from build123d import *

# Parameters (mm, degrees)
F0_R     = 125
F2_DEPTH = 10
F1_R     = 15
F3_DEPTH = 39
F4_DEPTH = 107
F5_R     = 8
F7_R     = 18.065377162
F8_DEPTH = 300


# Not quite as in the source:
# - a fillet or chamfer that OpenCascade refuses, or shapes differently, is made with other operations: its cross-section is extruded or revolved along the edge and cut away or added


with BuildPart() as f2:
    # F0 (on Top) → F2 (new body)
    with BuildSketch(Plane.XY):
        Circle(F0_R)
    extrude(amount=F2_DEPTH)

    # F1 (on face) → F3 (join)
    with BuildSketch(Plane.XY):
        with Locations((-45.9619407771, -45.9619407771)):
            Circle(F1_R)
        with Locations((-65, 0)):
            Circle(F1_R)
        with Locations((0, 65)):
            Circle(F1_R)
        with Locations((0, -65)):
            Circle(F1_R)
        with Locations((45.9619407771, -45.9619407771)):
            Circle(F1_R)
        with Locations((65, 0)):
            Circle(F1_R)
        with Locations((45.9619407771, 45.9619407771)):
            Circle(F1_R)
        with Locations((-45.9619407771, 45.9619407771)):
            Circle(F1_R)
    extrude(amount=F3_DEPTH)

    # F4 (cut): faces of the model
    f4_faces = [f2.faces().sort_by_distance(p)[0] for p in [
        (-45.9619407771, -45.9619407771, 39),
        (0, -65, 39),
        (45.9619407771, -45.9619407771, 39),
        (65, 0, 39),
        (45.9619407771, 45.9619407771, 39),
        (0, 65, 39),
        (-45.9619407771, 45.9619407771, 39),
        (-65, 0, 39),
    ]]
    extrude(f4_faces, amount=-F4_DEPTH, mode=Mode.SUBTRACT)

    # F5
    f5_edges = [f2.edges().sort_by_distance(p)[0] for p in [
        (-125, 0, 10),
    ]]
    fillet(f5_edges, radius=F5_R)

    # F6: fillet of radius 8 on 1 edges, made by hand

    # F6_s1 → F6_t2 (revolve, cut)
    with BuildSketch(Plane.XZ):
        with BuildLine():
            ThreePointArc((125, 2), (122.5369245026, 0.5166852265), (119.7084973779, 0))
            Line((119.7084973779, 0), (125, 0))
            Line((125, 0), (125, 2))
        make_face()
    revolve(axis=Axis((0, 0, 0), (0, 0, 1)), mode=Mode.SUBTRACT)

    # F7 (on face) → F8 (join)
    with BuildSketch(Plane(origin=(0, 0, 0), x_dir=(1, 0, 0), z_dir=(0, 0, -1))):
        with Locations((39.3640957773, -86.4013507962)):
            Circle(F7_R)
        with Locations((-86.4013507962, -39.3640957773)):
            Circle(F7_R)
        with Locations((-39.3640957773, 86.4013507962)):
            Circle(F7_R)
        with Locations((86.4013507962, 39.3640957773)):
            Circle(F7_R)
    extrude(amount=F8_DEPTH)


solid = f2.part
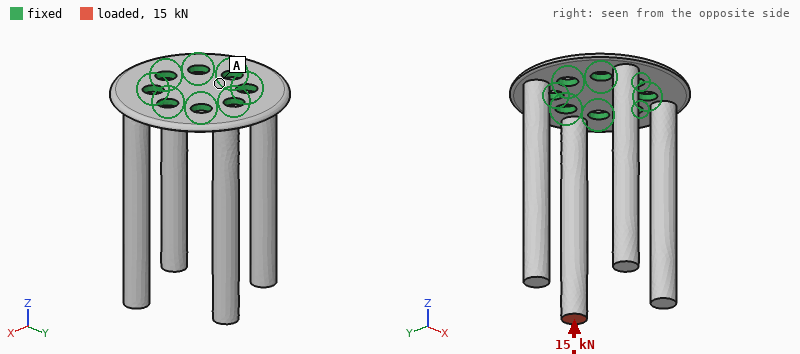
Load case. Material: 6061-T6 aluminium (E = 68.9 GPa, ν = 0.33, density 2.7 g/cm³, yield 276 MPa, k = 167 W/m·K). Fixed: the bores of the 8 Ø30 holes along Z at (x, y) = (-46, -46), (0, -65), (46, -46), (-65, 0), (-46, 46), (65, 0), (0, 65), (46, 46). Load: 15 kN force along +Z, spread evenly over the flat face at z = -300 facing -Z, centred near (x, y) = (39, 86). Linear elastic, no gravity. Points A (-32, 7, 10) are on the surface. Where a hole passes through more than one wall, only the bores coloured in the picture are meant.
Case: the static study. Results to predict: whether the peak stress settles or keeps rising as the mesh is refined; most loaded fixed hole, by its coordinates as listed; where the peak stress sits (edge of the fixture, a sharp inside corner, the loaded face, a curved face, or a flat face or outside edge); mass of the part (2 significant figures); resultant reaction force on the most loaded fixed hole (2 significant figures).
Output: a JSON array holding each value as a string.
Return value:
["keeps rising", "(46, 46)", "edge of the fixture", "4.5 kg", "8.9 kN"]
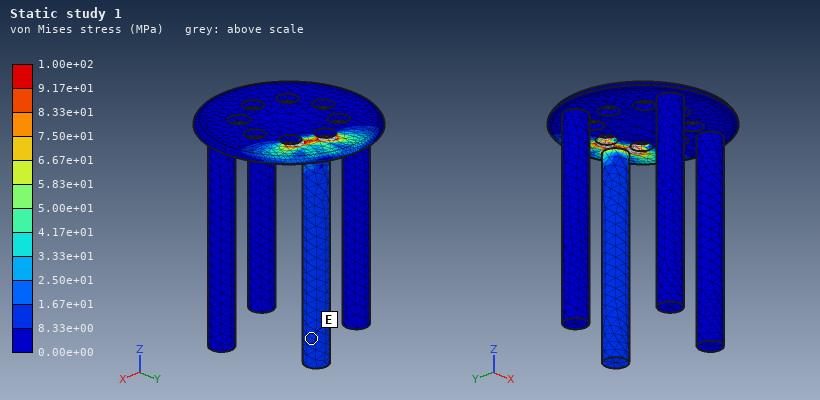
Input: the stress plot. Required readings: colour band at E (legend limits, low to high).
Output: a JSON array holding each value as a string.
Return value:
["8.33e+00 to 1.67e+01 MPa"]
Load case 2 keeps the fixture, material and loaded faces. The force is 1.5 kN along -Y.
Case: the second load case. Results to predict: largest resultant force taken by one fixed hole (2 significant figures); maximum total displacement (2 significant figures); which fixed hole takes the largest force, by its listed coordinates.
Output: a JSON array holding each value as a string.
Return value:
["5.6 kN", "5.4 mm", "(0, 65)"]
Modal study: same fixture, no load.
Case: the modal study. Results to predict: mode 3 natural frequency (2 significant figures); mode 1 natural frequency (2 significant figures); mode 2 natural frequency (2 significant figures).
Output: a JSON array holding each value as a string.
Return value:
["160 Hz", "160 Hz", "160 Hz"]
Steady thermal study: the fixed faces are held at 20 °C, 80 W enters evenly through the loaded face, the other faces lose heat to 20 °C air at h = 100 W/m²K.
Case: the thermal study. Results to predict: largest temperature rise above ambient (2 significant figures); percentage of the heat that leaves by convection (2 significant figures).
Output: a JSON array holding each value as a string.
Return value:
["57 K", "87 %"]
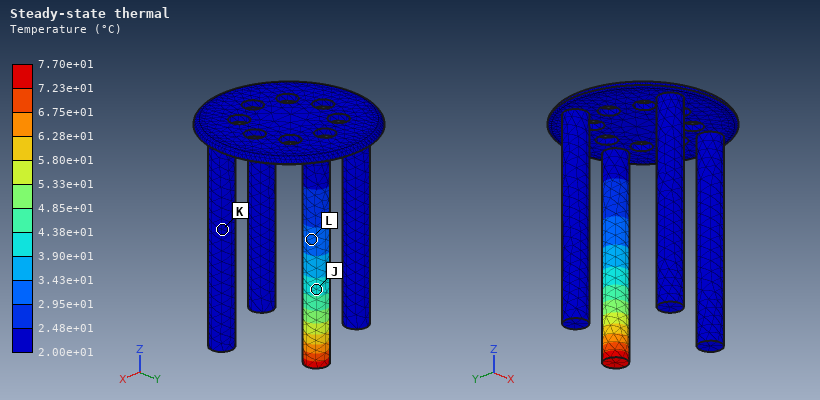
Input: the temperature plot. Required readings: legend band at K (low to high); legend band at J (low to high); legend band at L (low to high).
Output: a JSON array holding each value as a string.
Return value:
["2.00e+01 to 2.48e+01 °C", "3.90e+01 to 4.38e+01 °C", "2.95e+01 to 3.43e+01 °C"]
